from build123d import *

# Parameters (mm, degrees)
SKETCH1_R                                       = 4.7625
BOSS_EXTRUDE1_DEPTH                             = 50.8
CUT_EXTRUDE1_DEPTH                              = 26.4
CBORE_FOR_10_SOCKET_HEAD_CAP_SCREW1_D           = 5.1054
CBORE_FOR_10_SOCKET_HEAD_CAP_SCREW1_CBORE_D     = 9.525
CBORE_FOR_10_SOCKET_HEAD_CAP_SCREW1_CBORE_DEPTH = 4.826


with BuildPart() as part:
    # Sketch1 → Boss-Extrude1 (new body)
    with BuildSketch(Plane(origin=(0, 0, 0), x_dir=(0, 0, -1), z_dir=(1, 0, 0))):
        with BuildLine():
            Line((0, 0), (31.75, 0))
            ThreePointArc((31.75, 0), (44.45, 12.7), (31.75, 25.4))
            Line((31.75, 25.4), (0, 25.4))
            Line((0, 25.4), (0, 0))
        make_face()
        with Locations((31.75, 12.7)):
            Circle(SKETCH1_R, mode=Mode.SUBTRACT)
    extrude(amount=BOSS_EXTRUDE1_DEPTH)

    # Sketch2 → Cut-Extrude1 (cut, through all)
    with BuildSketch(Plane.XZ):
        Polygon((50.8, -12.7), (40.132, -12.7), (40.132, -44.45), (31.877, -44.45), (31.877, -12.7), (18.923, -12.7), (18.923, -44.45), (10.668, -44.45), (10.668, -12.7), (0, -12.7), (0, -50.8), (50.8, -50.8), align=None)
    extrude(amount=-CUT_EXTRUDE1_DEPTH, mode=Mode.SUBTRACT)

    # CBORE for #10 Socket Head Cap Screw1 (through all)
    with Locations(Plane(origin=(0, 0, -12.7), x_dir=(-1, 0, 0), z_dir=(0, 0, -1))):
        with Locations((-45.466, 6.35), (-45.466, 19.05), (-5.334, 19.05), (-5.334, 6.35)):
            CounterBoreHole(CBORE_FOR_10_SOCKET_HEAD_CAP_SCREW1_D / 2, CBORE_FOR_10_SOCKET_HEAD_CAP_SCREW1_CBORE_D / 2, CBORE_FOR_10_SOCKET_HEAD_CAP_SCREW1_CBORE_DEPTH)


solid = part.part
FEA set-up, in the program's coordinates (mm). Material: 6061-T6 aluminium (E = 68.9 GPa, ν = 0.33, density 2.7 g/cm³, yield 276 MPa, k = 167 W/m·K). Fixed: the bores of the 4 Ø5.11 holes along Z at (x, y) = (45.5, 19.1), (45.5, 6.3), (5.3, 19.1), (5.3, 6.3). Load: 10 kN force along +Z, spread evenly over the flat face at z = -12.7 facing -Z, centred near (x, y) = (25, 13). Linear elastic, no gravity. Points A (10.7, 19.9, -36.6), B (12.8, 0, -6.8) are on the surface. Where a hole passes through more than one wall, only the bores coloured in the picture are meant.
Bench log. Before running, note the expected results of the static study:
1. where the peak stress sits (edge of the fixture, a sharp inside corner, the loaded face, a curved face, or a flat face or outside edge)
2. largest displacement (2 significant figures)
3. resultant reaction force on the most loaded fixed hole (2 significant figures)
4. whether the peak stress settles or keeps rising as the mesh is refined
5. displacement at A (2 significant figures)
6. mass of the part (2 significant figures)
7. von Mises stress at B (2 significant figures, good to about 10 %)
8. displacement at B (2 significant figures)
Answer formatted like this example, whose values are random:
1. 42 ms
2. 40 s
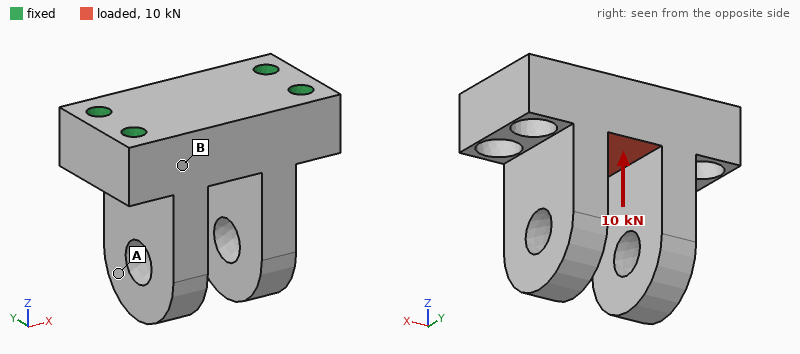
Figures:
1. edge of the fixture
2. 60 µm
3. 2.9 kN
4. keeps rising
5. 45 µm
6. 68 g
7. 39 MPa
8. 11 µm
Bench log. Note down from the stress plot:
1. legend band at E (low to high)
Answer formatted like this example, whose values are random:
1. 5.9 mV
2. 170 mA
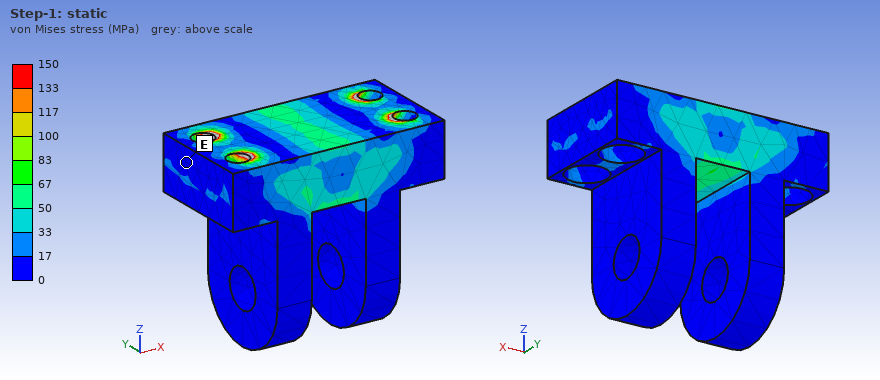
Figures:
1. 0 to 17 MPa
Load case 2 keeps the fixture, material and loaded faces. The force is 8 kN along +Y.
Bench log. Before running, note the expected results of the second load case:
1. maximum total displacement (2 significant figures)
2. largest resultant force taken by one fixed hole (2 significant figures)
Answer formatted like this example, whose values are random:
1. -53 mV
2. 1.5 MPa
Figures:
1. 39 µm
2. 3.3 kN
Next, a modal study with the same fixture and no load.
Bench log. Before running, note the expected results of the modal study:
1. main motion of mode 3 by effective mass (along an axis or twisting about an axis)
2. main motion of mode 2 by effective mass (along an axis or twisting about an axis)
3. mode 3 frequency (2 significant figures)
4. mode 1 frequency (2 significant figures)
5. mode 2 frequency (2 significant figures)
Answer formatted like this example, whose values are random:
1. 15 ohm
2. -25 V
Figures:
1. along Y
2. along X
3. 8200 Hz
4. 5900 Hz
5. 6500 Hz
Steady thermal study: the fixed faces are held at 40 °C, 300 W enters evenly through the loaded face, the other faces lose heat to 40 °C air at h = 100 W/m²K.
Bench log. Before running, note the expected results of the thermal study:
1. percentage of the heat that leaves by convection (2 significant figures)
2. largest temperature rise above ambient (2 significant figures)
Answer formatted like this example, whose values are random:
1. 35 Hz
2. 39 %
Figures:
1. 6.8 %
2. 66 K
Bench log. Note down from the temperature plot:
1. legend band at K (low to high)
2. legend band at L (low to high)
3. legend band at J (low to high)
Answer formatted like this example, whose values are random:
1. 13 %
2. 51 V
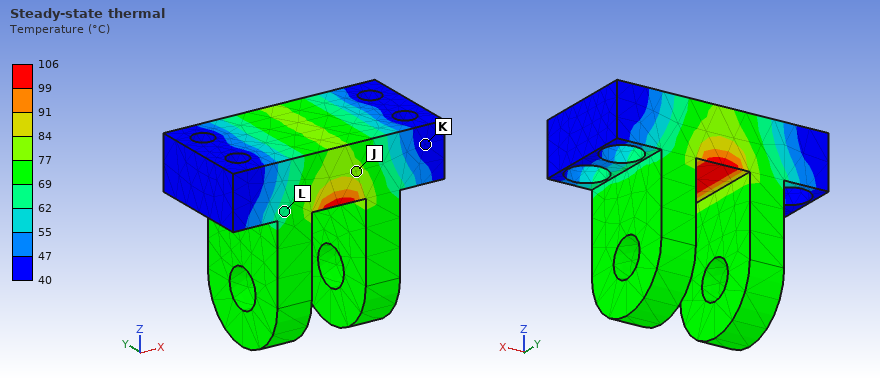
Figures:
1. 40 to 47 °C
2. 62 to 69 °C
3. 77 to 84 °C
